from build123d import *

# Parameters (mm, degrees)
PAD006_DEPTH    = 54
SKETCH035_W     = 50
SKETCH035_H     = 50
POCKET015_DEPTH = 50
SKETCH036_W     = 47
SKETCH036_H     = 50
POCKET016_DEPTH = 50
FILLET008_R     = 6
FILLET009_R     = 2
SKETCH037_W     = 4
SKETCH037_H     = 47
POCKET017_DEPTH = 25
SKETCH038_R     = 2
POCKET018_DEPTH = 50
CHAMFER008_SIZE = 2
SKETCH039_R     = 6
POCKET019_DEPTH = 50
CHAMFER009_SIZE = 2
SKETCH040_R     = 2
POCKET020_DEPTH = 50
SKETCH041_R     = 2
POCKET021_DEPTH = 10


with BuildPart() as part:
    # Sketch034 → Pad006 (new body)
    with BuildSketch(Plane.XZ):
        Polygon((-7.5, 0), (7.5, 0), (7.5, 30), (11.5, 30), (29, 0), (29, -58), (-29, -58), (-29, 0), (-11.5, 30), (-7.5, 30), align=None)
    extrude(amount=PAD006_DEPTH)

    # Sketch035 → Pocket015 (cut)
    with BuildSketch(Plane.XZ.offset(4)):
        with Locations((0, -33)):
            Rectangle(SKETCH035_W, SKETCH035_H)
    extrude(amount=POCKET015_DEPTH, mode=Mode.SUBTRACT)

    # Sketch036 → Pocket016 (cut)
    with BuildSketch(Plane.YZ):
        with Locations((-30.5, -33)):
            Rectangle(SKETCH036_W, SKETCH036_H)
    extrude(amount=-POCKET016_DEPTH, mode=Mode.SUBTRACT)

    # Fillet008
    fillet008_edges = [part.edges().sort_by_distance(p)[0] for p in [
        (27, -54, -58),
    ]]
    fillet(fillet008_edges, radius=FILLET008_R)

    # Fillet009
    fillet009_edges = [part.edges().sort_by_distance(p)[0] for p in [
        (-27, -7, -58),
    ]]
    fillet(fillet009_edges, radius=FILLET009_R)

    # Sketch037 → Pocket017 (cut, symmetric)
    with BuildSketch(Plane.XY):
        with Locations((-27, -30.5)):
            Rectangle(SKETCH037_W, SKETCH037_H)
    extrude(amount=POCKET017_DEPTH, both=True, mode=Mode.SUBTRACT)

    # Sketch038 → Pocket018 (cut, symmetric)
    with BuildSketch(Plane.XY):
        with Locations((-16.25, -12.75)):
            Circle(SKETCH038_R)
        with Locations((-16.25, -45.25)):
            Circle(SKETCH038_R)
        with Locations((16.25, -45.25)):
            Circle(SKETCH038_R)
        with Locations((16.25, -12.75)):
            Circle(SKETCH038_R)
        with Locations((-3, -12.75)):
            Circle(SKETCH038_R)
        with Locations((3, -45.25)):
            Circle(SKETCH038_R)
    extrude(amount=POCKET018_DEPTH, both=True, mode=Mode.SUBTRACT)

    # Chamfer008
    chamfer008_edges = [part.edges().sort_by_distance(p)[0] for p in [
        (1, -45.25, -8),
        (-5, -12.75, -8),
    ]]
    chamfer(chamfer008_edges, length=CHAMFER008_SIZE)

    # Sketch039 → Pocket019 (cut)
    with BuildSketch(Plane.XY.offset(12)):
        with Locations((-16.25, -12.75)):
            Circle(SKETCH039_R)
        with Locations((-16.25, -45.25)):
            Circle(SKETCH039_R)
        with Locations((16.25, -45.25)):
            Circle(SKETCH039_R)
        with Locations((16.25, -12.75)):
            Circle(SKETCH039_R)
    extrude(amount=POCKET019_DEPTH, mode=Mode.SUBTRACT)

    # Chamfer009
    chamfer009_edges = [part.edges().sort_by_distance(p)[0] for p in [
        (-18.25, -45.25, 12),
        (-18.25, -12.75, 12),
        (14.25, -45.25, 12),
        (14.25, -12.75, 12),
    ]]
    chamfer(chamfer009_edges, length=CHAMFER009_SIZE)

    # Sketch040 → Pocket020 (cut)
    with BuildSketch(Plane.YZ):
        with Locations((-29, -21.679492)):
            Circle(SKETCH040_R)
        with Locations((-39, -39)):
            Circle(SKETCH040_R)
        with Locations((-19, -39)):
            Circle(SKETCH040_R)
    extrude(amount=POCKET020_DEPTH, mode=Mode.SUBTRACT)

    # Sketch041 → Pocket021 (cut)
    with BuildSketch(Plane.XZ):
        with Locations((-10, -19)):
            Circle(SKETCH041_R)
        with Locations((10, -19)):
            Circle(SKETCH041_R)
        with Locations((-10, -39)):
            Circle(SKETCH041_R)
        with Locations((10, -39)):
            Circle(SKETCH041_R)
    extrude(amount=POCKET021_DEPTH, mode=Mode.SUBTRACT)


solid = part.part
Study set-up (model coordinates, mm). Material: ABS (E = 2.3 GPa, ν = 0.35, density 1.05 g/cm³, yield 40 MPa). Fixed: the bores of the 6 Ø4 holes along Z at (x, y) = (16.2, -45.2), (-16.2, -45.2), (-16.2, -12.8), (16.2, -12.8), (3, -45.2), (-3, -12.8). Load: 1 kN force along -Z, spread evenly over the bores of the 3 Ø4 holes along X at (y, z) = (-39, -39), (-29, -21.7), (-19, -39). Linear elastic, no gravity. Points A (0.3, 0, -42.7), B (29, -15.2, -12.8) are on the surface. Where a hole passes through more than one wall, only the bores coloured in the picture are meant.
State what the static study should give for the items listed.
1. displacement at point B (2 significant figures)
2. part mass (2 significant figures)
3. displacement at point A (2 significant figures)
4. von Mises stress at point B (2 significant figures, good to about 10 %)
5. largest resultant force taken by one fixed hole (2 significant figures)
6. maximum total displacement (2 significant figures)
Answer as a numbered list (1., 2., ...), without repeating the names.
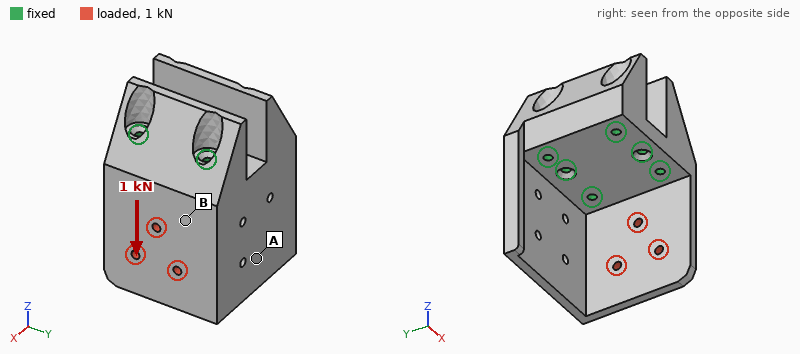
1. 0.054 mm
2. 84 g
3. 0.059 mm
4. 3.7 MPa
5. 540 N
6. 0.19 mm
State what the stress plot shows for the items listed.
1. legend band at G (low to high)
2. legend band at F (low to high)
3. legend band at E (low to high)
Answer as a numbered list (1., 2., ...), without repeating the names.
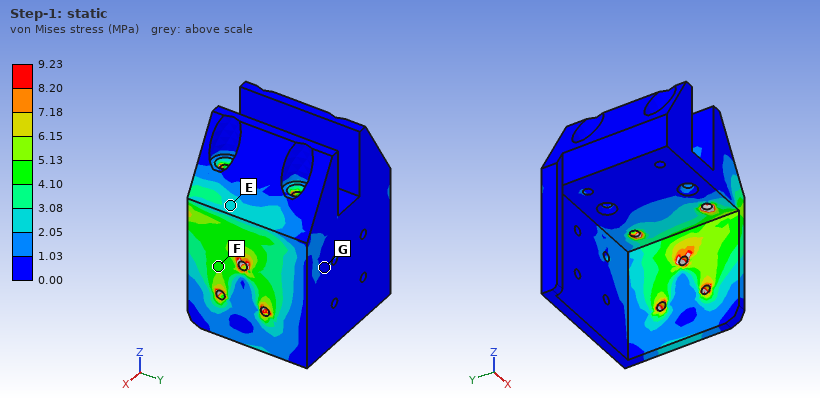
1. 0.00 to 1.03 MPa
2. 4.10 to 5.13 MPa
3. 2.05 to 3.08 MPa
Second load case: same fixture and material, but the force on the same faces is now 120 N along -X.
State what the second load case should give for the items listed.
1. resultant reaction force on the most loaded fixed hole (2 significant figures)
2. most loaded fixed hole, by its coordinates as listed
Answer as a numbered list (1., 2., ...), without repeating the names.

1. 74 N
2. (16.2, -12.8)
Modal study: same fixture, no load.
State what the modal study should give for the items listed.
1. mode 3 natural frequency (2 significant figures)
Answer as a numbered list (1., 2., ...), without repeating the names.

1. 1700 Hz
